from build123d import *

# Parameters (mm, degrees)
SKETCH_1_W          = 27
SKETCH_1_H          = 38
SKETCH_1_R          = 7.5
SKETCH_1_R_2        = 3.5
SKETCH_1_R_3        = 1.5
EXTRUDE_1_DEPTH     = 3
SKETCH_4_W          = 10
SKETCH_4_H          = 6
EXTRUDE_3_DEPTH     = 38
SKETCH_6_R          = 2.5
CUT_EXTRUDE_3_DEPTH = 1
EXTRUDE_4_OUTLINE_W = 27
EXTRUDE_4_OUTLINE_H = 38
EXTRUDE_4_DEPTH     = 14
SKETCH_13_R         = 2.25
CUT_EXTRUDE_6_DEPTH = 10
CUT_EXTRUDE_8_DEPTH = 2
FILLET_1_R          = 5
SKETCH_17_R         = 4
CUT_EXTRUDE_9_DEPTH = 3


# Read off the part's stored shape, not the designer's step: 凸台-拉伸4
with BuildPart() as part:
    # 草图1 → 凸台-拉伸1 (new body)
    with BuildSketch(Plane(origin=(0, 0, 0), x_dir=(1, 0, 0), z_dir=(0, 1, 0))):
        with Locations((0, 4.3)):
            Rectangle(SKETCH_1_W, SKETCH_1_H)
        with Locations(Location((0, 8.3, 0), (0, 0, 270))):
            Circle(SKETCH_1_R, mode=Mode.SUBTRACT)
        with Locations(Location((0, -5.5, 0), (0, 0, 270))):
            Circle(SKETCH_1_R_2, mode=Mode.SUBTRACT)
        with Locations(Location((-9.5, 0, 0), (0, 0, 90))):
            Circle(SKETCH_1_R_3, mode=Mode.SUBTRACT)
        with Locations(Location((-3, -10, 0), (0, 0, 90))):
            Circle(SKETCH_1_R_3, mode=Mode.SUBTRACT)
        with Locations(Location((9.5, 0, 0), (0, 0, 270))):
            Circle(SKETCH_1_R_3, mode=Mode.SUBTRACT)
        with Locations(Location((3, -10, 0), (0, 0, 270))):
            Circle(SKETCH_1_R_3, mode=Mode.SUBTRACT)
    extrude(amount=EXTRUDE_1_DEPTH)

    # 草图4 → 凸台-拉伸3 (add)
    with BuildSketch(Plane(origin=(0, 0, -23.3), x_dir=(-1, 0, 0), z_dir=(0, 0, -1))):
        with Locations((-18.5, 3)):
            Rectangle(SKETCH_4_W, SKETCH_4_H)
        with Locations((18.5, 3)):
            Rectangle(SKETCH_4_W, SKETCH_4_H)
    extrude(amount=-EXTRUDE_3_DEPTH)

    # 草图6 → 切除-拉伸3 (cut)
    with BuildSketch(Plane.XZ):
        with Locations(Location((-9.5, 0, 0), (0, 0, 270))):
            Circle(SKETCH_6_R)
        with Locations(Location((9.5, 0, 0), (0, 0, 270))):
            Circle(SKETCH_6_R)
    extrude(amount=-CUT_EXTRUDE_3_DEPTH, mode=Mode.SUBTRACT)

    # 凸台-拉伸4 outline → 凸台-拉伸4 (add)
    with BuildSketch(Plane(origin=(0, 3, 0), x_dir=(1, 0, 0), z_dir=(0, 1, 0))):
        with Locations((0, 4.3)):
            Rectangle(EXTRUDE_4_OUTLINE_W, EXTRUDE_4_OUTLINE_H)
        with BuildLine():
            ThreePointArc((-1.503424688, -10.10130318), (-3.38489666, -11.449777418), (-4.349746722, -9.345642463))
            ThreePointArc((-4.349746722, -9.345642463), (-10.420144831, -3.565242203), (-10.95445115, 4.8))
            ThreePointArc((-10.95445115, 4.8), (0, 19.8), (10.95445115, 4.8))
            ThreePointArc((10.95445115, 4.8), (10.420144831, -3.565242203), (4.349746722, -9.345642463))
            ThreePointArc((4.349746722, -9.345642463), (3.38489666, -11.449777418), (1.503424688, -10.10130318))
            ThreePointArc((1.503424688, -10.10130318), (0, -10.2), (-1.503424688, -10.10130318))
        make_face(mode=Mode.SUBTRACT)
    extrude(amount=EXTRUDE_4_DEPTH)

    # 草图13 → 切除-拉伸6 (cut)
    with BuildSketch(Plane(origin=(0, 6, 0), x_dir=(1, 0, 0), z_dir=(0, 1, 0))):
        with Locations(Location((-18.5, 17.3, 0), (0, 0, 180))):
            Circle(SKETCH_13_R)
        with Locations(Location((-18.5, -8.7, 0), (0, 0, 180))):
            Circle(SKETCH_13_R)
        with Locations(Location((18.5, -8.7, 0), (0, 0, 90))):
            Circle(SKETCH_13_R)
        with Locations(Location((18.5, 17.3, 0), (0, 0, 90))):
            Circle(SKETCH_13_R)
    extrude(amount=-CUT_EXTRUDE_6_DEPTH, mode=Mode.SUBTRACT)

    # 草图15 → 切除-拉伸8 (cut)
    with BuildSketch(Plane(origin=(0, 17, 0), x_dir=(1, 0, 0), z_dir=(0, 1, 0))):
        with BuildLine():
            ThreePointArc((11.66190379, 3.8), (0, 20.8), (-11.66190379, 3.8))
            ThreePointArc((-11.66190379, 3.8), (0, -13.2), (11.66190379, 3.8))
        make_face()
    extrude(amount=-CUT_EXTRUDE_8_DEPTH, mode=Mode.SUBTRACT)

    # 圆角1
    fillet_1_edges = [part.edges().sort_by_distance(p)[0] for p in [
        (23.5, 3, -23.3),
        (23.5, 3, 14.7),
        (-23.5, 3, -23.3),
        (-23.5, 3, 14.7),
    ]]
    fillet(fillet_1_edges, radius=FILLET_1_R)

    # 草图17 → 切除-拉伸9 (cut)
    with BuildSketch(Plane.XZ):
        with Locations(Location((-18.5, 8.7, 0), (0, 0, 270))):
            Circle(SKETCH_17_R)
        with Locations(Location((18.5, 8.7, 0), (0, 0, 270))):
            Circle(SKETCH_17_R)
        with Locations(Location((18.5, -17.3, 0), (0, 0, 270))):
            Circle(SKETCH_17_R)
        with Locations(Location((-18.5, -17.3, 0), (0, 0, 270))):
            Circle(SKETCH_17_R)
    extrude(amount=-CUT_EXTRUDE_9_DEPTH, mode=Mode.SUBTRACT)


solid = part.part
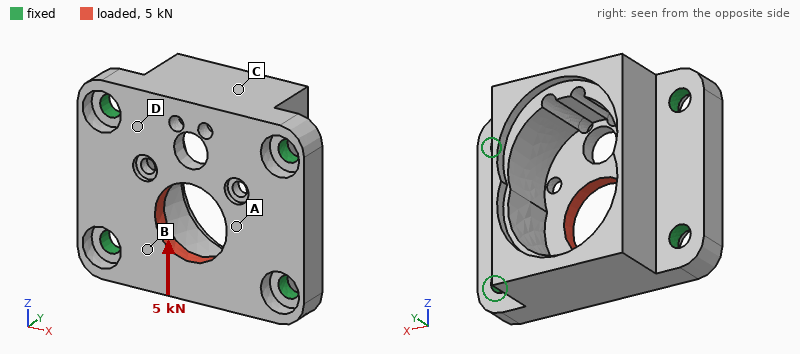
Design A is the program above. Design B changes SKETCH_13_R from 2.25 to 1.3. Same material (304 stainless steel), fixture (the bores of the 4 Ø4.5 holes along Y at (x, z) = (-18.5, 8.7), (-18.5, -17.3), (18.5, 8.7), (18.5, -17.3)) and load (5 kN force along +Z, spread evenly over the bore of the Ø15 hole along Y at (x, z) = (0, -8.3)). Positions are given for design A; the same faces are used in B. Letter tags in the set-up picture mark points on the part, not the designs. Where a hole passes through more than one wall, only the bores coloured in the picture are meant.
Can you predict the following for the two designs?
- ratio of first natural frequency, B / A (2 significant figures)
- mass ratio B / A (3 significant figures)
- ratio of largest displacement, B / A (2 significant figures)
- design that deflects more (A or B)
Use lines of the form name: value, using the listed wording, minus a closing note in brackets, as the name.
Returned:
ratio of first natural frequency, B / A: 0.85
mass ratio B / A: 1.01
ratio of largest displacement, B / A: 1.1
design that deflects more: B
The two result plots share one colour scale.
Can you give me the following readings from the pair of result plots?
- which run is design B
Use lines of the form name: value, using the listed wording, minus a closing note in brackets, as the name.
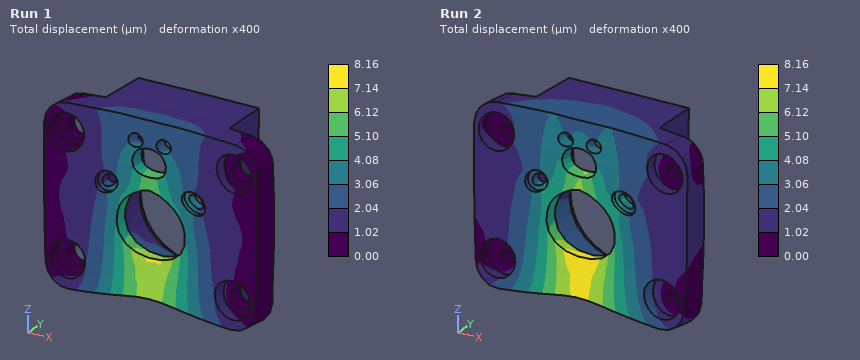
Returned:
which run is design B: Run 2
